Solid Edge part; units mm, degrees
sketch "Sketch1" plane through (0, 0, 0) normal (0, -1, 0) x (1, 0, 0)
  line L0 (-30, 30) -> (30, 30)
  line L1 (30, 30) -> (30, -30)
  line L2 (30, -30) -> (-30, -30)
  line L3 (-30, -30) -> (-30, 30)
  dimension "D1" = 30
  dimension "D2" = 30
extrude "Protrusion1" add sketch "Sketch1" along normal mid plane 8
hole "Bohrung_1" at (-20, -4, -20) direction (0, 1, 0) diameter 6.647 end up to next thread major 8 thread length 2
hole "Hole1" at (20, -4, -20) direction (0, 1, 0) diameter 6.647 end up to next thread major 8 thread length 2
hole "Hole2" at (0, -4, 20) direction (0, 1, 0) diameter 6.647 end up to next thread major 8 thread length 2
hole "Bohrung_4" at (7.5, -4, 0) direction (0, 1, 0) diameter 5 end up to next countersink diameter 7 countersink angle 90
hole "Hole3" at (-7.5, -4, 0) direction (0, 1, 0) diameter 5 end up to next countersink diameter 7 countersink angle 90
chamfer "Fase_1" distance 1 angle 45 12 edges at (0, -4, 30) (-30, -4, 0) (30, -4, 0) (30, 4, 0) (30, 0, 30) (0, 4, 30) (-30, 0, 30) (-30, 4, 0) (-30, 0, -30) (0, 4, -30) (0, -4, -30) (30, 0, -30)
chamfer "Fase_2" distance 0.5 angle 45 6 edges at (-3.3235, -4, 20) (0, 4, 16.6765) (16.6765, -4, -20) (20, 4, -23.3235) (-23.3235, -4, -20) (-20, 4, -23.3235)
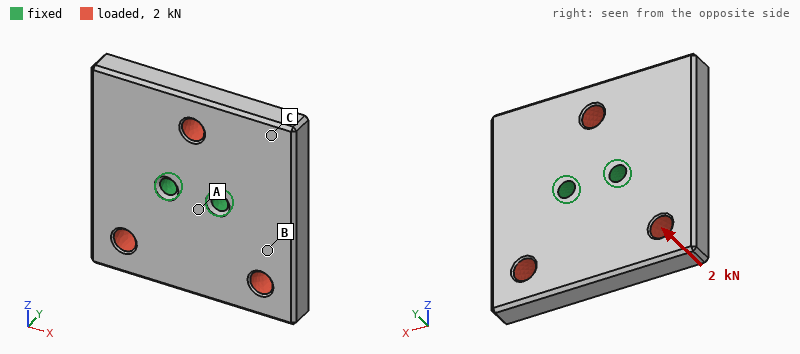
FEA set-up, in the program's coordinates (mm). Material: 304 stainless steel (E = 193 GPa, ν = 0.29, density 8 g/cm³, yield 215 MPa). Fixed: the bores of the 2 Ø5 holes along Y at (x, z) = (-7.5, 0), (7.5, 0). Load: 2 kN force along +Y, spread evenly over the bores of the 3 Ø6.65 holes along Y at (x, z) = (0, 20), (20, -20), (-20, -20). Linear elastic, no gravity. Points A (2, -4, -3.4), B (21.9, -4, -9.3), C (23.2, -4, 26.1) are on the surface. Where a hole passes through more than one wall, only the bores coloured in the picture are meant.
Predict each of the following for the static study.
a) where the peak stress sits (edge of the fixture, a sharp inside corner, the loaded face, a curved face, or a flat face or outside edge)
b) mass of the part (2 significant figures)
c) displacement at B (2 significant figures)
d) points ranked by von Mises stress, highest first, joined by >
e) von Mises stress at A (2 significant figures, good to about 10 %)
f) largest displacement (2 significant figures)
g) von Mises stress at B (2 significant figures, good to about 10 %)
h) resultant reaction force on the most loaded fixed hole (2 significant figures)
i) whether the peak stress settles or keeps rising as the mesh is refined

edge of the fixture
220 g
6.0 µm
A > B > C
31 MPa
20 µm
18 MPa
1.0 kN
keeps rising
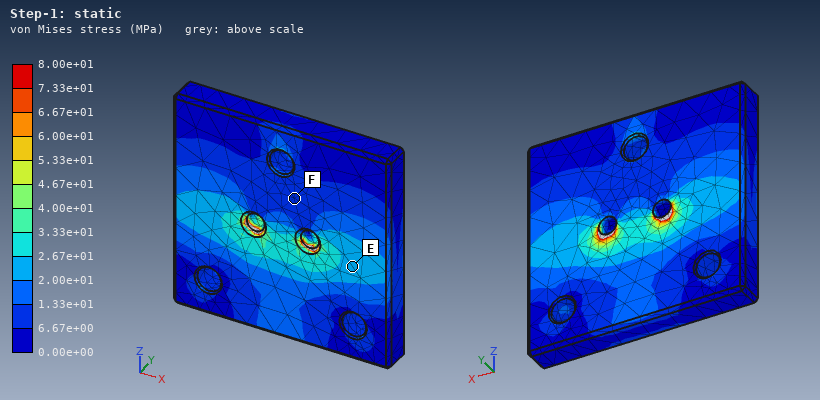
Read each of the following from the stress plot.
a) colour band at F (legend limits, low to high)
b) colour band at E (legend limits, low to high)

6.67e+00 to 1.33e+01 MPa
2.00e+01 to 2.67e+01 MPa
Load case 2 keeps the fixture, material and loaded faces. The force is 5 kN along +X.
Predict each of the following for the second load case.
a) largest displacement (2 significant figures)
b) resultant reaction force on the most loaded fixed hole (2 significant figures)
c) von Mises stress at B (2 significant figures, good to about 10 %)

6.7 µm
3.0 kN
9.1 MPa
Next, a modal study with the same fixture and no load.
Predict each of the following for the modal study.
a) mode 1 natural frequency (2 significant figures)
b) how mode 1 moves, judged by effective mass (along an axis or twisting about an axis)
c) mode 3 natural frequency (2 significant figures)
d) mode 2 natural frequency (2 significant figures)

5000 Hz
twisting about X
6800 Hz
6700 Hz
